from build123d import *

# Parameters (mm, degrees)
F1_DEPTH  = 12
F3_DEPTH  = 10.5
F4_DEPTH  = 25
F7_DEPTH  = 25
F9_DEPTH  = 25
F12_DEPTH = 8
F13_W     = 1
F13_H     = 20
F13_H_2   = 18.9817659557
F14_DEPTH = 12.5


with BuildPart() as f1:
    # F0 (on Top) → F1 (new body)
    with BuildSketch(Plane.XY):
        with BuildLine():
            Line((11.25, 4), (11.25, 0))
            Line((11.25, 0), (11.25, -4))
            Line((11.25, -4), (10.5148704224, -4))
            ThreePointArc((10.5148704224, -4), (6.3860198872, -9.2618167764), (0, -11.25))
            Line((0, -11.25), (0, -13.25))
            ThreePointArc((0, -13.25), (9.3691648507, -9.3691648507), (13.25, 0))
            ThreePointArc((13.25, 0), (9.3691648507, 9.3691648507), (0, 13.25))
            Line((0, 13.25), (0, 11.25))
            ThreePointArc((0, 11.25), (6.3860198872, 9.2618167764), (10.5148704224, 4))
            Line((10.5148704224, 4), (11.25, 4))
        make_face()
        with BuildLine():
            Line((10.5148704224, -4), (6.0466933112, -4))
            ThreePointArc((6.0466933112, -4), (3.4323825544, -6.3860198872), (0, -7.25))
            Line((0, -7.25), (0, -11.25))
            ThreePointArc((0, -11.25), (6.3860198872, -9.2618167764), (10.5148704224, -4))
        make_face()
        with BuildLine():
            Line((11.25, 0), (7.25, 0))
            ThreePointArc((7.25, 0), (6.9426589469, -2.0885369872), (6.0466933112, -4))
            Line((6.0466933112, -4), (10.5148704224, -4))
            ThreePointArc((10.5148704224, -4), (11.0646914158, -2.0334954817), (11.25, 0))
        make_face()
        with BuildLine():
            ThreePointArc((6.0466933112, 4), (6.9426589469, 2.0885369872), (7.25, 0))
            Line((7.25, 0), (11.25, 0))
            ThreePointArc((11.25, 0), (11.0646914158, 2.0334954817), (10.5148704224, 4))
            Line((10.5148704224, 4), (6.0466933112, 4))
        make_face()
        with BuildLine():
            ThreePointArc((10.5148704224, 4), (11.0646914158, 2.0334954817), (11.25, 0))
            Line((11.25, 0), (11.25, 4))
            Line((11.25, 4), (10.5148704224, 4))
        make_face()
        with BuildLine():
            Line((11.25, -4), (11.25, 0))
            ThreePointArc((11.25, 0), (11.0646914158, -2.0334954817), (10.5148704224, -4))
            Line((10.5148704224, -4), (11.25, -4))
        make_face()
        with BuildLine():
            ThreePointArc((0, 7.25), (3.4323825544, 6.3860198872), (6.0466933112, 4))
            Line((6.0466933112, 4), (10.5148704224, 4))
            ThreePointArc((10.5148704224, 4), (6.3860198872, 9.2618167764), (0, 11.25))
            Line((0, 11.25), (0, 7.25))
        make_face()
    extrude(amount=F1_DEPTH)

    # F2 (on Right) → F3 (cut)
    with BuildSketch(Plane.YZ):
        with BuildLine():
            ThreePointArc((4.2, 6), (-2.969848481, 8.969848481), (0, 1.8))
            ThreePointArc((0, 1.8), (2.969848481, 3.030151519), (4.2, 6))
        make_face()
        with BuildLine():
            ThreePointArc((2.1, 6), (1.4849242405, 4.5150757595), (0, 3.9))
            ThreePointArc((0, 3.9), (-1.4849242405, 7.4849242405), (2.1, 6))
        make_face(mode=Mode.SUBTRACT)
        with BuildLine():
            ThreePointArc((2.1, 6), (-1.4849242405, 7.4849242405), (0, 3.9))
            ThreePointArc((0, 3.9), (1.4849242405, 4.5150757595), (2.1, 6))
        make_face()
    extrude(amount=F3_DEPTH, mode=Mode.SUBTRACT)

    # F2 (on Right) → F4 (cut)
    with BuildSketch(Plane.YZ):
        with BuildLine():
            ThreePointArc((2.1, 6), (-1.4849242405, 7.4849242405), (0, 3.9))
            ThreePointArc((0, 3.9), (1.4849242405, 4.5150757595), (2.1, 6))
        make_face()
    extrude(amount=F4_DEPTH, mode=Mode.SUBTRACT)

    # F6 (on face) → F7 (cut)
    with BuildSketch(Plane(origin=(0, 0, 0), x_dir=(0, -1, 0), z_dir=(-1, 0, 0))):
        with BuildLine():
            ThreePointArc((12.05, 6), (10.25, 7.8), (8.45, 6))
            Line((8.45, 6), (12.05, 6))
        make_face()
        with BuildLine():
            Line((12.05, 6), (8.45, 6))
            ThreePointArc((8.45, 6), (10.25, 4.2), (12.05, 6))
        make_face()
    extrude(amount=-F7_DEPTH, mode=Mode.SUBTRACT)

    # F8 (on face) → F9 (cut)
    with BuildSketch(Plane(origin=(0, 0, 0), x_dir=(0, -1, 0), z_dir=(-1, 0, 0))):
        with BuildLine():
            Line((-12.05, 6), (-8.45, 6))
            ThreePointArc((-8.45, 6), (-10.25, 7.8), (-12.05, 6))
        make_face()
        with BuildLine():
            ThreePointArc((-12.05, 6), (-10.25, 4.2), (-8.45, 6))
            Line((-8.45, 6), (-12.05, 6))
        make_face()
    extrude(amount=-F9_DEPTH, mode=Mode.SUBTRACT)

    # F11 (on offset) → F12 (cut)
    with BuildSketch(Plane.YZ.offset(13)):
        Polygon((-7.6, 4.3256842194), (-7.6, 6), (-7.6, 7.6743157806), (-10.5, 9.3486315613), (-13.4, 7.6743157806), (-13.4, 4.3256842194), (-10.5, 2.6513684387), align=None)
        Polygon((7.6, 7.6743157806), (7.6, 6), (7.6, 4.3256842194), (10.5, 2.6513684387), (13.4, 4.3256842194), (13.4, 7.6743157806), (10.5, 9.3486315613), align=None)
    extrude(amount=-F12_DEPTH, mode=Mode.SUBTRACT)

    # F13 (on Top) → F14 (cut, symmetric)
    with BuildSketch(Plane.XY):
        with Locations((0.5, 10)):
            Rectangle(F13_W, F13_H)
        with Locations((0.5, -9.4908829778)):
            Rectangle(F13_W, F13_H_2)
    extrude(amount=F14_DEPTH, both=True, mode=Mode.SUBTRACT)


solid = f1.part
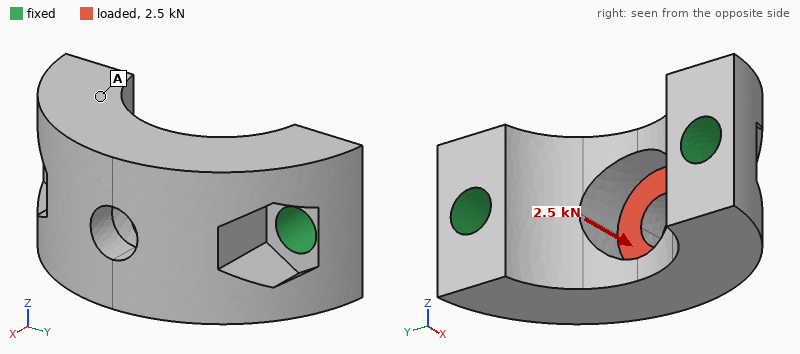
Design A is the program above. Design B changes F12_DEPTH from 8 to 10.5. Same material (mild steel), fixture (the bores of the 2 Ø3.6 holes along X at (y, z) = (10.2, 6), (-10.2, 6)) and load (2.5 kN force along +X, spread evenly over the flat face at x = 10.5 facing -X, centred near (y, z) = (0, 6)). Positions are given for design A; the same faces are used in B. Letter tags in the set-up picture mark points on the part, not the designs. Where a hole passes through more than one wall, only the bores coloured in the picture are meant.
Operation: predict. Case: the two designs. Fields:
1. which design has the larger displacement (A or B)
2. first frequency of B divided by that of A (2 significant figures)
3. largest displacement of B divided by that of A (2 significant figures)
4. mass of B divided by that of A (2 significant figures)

B
0.42
1.3
0.95
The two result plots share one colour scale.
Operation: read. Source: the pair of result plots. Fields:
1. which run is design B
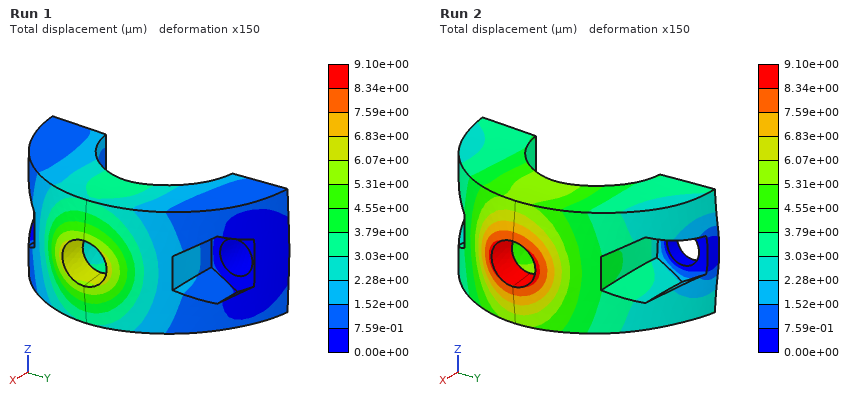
Run 2
